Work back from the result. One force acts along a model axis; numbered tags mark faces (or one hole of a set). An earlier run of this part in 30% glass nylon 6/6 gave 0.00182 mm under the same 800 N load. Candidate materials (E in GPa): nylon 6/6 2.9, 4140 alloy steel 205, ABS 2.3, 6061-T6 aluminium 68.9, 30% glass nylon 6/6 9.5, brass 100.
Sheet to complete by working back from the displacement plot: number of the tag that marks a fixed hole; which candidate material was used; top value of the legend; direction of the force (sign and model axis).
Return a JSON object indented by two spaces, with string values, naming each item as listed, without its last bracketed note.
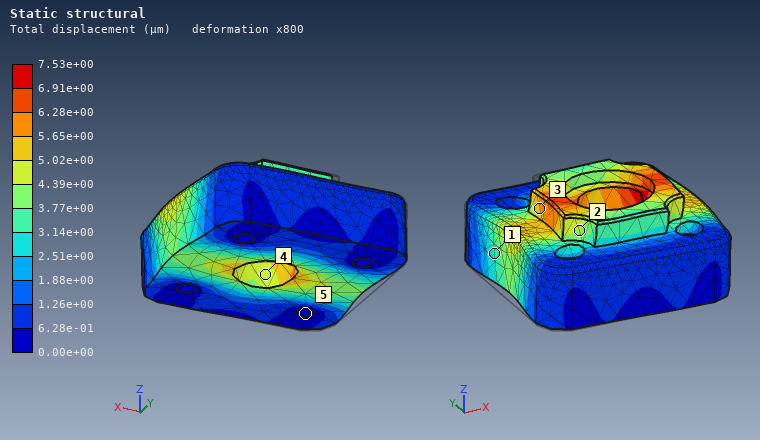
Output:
{
  "number of the tag that marks a fixed hole": "5",
  "which candidate material was used": "ABS",
  "top value of the legend": "7.53e+00 µm",
  "direction of the force": "+X"
}
